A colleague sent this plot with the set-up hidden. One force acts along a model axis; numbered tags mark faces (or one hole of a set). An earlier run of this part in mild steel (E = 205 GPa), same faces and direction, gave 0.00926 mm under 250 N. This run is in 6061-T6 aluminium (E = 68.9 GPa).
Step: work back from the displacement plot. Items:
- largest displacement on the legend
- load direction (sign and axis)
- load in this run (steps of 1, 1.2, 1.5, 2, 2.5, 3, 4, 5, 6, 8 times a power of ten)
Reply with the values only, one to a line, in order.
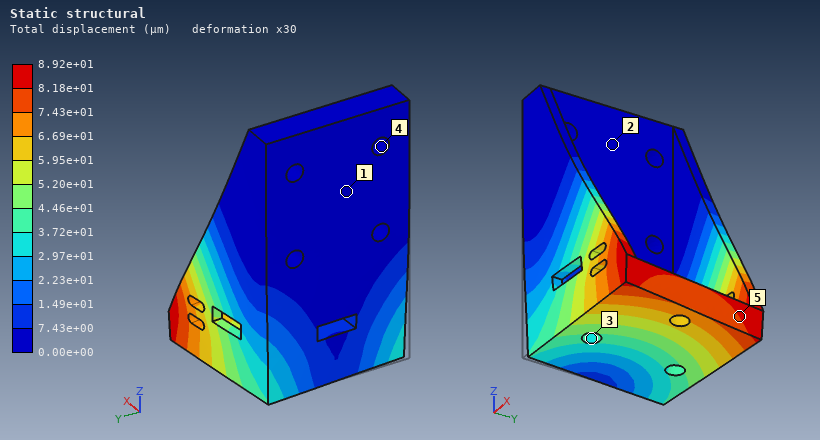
8.92e+01 µm
+Y
800 N
